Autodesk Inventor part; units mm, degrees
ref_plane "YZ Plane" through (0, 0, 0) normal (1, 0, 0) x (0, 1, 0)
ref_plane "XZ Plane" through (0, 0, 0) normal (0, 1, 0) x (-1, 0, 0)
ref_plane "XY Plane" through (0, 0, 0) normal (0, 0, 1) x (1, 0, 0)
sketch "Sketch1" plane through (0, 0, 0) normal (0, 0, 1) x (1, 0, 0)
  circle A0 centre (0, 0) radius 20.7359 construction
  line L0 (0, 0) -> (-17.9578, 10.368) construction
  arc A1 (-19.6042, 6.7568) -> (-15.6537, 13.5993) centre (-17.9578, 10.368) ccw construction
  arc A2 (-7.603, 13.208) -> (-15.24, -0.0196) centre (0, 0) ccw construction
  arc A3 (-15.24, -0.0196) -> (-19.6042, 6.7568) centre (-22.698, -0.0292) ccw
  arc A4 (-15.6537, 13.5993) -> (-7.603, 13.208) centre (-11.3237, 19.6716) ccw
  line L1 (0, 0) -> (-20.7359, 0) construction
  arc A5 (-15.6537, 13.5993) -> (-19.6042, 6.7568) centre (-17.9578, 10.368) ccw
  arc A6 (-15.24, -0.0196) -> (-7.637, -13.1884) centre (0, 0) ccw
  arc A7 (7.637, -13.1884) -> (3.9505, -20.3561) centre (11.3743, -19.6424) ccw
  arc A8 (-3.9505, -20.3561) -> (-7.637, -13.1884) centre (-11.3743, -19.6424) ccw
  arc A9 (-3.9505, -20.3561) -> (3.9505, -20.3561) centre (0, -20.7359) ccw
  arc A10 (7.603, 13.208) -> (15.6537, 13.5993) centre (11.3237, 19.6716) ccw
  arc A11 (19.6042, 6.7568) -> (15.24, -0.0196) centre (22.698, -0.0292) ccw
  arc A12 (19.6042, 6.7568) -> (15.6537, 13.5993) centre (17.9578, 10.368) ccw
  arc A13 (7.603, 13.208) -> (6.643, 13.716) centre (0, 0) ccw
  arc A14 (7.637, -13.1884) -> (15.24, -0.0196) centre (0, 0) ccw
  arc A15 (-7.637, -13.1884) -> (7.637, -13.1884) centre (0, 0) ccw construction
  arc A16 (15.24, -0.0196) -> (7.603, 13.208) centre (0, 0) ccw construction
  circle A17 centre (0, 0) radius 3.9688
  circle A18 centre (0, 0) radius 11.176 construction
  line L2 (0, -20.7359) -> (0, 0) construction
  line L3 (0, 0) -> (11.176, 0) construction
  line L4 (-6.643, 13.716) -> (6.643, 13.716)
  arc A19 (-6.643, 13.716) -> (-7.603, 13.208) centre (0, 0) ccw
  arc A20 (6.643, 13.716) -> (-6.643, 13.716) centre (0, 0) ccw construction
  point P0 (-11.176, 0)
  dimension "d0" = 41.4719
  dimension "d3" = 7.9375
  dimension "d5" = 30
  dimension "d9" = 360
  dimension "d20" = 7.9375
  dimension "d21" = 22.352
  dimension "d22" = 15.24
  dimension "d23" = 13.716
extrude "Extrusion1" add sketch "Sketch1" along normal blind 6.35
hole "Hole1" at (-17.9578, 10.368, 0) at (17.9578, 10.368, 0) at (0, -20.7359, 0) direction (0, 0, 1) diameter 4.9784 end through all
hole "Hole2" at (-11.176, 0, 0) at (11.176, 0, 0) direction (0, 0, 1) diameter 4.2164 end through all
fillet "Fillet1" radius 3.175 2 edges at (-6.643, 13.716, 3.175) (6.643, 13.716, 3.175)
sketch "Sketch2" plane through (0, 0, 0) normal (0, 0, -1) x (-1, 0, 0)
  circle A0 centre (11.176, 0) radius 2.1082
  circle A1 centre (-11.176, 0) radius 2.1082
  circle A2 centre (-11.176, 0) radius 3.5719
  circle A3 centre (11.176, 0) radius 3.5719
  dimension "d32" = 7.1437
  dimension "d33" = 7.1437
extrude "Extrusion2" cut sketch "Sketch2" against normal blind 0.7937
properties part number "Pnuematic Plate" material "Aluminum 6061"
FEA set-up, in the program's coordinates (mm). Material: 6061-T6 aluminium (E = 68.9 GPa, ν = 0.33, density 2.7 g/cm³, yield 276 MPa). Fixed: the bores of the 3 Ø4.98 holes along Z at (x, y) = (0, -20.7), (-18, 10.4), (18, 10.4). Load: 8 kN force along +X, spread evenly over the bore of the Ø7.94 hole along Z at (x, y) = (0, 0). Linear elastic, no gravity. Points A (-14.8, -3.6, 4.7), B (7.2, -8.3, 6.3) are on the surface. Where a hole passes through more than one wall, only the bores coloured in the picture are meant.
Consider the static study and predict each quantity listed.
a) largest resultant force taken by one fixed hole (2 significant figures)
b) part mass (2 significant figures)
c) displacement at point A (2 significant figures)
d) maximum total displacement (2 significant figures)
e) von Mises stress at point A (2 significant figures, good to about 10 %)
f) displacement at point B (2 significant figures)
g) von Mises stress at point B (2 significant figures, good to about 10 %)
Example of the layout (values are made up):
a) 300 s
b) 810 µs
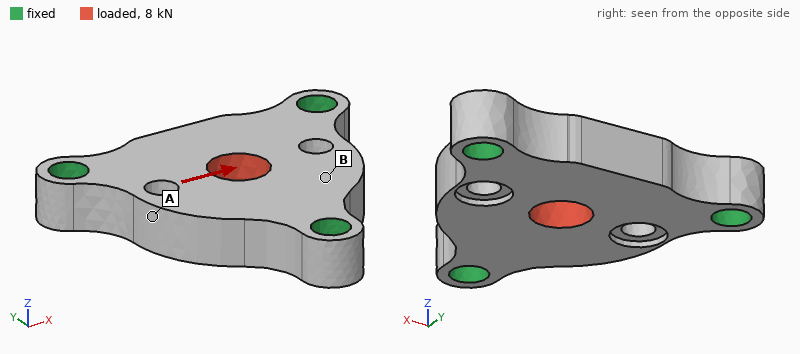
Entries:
a) 3.3 kN
b) 14 g
c) 19 µm
d) 25 µm
e) 58 MPa
f) 19 µm
g) 27 MPa
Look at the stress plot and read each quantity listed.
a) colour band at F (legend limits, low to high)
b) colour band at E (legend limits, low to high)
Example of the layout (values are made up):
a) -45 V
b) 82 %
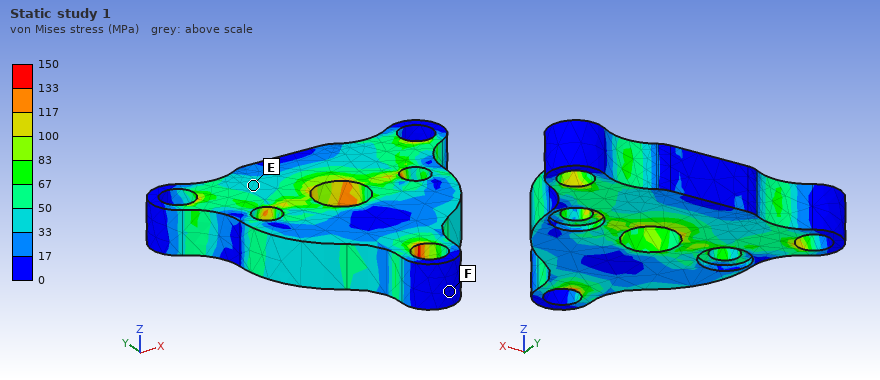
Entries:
a) 0 to 17 MPa
b) 33 to 50 MPa
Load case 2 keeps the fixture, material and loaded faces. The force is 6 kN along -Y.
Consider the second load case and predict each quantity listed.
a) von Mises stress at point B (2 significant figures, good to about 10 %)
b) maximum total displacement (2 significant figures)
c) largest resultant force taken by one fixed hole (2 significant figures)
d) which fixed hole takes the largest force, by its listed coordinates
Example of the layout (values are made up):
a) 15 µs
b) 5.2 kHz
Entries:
a) 27 MPa
b) 19 µm
c) 3.2 kN
d) (0, -20.7)
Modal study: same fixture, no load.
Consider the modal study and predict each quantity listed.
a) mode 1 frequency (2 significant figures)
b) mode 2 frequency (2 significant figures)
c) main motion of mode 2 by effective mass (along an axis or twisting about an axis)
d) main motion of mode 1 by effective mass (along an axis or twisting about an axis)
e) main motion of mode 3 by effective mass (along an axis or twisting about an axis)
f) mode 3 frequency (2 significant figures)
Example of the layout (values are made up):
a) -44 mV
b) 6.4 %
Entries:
a) 20 kHz
b) 24 kHz
c) twisting about Y
d) along Z
e) twisting about X
f) 27 kHz
